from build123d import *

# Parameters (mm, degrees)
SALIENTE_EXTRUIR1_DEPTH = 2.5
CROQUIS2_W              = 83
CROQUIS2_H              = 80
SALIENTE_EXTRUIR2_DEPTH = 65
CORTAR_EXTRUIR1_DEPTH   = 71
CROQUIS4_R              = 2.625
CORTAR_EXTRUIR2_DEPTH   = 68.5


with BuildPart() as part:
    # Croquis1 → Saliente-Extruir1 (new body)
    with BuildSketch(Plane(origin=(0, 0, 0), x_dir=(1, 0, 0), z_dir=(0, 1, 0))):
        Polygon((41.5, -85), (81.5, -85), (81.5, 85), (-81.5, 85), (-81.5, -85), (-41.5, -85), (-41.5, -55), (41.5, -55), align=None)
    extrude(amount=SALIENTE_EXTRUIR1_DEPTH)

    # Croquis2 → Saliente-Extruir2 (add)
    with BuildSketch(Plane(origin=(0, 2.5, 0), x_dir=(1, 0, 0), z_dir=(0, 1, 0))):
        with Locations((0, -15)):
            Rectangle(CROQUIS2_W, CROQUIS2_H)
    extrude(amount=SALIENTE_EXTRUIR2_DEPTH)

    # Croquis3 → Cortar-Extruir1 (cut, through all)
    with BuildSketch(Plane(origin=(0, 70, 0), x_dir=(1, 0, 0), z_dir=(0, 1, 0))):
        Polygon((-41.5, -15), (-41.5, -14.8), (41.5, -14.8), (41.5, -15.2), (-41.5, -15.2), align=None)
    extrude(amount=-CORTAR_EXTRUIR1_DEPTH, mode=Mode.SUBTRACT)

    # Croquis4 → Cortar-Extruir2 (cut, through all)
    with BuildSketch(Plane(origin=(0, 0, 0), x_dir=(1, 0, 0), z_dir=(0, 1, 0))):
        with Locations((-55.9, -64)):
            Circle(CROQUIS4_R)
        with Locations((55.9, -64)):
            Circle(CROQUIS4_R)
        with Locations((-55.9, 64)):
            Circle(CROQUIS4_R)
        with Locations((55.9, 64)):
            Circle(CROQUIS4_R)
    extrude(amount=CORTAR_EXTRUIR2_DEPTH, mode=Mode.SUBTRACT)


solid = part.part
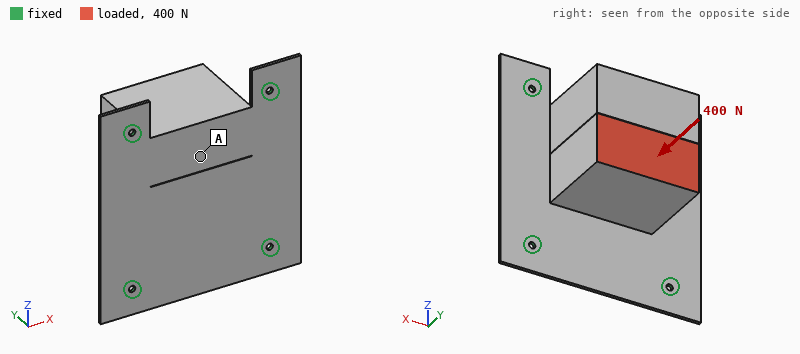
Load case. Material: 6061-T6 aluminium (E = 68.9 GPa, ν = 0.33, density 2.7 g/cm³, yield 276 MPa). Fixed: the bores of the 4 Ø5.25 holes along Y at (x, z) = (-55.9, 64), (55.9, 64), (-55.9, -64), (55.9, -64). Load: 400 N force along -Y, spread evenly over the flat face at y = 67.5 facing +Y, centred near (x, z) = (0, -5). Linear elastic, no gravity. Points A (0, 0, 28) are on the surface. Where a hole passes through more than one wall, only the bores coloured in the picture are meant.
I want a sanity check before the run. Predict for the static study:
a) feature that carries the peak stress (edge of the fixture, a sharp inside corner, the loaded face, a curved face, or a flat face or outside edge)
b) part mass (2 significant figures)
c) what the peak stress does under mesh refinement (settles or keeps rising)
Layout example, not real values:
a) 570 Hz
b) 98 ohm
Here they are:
a) a sharp inside corner
b) 1.3 kg
c) keeps rising
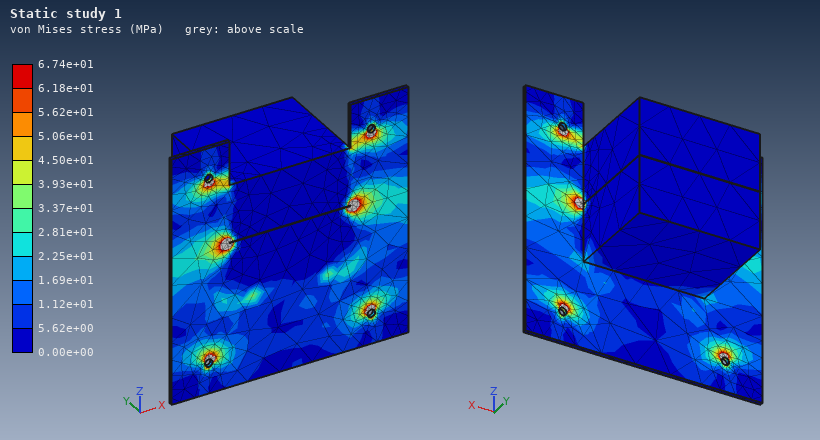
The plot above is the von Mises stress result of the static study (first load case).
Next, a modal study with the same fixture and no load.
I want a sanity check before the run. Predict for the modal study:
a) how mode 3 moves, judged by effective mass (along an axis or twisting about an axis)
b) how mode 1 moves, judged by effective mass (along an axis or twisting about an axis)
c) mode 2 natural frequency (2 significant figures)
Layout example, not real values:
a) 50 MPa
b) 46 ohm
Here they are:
a) along X
b) along Y
c) 330 Hz
